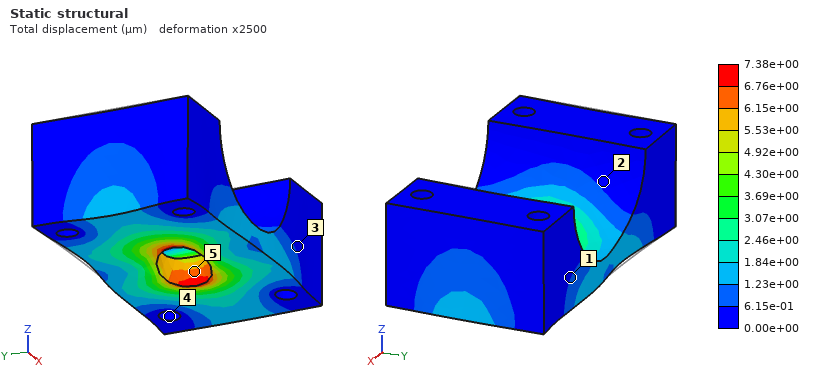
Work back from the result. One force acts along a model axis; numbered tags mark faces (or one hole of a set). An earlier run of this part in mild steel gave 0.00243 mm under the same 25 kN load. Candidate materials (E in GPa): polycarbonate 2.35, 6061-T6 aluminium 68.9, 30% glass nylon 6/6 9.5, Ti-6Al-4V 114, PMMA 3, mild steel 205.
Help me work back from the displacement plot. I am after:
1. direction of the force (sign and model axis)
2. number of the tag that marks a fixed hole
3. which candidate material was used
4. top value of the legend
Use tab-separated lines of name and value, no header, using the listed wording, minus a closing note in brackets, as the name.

direction of the force	+X
number of the tag that marks a fixed hole	4
which candidate material was used	6061-T6 aluminium
top value of the legend	7.38e+00 µm
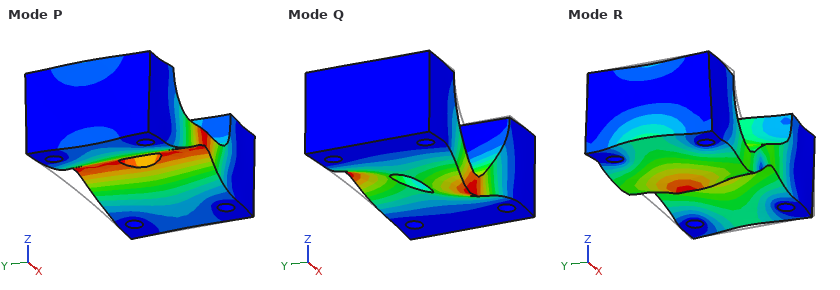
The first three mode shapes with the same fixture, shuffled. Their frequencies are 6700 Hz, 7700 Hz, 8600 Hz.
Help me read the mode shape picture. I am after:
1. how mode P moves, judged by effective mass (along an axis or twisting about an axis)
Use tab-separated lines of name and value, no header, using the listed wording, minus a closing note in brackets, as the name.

how mode P moves, judged by effective mass	along Z
